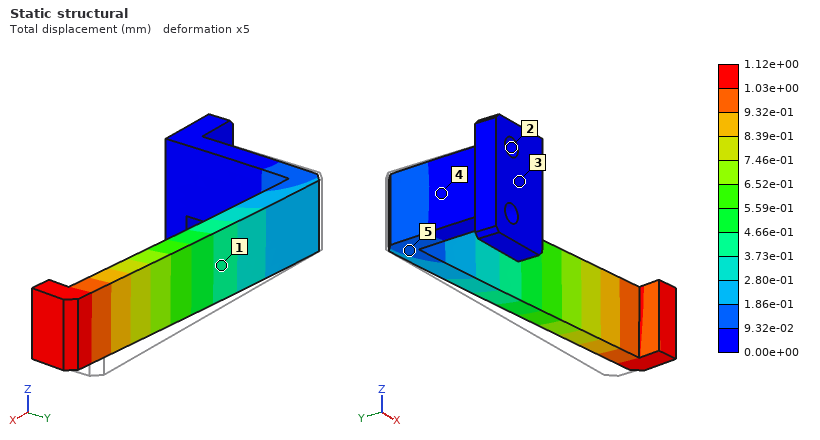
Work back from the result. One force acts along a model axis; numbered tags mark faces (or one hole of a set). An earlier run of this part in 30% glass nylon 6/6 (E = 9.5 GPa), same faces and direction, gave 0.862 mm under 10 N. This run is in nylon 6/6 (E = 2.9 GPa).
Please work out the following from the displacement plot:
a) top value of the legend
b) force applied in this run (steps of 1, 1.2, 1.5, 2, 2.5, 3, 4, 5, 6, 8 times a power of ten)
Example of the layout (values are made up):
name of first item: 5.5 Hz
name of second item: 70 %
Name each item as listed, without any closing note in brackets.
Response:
top value of the legend: 1.12e+00 mm
force applied in this run: 4 N
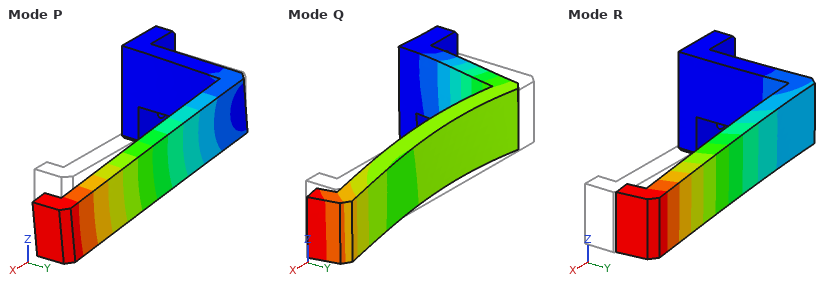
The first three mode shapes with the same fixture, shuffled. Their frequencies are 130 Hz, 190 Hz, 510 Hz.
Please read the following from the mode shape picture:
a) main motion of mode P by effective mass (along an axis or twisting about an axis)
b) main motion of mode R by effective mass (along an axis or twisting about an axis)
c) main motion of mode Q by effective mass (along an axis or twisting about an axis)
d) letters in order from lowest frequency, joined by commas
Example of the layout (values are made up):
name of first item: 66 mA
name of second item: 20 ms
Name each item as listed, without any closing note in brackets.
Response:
main motion of mode P by effective mass: along Z
main motion of mode R by effective mass: along Y
main motion of mode Q by effective mass: along X
letters in order from lowest frequency, joined by commas: R, P, Q
